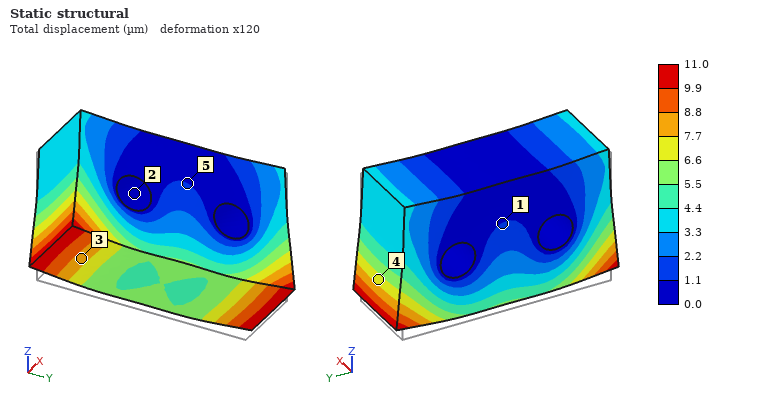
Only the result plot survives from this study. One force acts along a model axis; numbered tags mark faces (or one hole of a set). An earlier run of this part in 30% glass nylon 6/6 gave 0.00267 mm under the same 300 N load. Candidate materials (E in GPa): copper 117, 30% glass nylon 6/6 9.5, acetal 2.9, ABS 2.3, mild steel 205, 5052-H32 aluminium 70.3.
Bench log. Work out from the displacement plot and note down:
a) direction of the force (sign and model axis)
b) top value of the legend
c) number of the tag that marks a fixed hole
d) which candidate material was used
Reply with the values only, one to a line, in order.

+Z
11.0 µm
2
ABS
